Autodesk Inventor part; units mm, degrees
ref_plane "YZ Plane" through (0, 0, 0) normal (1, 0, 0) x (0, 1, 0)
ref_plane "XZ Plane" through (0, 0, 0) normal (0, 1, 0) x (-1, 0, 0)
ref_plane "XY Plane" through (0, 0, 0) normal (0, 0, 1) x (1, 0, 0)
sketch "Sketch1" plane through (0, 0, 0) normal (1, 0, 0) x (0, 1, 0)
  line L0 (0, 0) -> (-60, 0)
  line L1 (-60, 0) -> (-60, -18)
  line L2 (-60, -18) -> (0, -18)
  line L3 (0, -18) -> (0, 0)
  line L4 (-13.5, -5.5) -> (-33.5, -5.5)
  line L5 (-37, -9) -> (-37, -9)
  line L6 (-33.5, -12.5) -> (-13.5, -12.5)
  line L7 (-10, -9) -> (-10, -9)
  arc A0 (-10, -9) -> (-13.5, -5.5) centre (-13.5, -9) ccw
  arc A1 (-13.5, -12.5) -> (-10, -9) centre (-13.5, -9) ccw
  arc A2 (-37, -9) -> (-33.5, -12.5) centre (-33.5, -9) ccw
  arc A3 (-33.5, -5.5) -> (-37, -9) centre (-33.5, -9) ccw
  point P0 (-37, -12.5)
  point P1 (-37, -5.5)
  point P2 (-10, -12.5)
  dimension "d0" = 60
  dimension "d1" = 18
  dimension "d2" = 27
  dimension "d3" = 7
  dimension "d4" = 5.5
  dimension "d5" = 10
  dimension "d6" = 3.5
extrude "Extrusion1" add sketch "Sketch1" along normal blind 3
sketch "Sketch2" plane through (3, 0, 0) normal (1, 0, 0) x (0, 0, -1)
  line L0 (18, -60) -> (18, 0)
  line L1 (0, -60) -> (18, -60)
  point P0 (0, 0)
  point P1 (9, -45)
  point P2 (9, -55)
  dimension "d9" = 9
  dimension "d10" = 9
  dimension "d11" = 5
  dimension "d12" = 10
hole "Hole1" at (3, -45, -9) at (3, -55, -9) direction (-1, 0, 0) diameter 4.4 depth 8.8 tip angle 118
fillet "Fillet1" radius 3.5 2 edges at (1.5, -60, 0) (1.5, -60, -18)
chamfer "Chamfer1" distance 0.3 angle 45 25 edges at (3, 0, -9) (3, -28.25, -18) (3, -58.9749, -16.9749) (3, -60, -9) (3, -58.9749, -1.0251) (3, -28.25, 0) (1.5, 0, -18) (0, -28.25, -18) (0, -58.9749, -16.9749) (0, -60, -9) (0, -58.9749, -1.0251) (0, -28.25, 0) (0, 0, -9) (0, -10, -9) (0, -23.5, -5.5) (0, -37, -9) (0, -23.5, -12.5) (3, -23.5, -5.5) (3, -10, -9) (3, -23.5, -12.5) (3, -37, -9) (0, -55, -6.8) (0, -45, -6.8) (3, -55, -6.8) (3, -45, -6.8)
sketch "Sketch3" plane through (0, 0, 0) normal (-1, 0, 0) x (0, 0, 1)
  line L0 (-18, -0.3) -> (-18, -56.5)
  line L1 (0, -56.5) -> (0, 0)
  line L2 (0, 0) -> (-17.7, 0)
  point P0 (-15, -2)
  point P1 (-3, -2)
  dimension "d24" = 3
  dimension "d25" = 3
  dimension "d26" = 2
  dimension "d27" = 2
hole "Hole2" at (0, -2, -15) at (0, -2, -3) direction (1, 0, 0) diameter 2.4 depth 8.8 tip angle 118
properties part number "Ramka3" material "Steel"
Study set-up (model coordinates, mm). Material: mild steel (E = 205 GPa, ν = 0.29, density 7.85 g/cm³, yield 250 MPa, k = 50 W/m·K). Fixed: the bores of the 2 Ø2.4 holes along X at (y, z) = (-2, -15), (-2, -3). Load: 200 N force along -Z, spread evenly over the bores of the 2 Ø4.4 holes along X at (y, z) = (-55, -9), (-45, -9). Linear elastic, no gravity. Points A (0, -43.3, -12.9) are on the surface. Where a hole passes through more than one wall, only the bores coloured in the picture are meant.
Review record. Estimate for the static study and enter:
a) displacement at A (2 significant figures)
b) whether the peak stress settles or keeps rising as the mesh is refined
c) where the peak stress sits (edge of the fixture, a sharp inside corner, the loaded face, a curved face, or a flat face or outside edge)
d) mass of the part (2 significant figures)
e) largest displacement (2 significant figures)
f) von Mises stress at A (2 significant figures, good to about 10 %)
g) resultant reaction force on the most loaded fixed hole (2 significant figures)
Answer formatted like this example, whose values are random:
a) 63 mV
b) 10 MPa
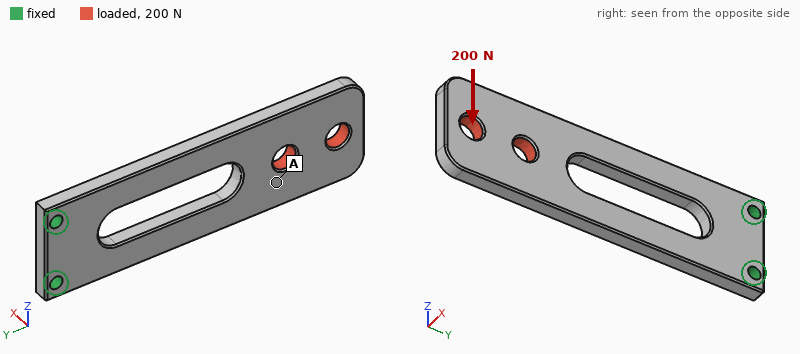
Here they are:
a) 47 µm
b) keeps rising
c) edge of the fixture
d) 20 g
e) 62 µm
f) 17 MPa
g) 730 N
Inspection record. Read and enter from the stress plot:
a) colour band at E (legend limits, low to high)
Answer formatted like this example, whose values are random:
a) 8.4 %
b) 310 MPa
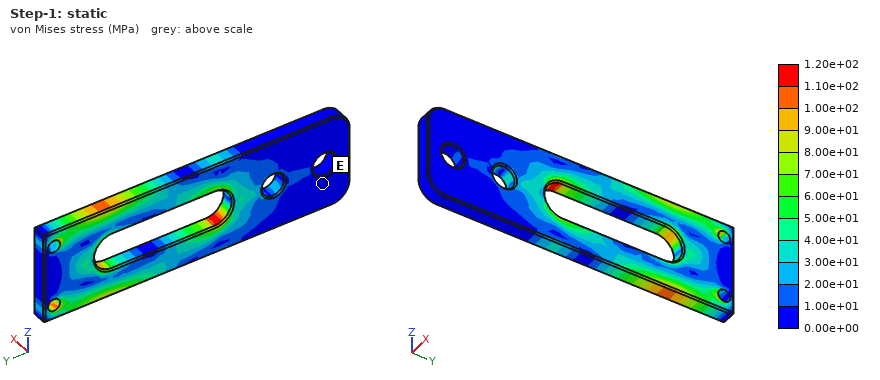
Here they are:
a) 0.00e+00 to 1.00e+01 MPa
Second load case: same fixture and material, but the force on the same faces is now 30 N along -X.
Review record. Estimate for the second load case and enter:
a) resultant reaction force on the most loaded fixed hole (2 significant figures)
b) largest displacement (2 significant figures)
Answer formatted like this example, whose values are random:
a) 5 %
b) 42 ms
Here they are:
a) 15 N
b) 0.25 mm
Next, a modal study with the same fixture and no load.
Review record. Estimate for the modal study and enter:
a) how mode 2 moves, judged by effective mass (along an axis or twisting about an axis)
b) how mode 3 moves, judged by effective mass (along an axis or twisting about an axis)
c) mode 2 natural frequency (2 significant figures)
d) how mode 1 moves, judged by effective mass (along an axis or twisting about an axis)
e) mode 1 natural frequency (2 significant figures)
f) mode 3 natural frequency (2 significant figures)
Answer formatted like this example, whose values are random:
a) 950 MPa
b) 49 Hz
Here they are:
a) along Z
b) twisting about Y
c) 3100 Hz
d) along X
e) 670 Hz
f) 3600 Hz
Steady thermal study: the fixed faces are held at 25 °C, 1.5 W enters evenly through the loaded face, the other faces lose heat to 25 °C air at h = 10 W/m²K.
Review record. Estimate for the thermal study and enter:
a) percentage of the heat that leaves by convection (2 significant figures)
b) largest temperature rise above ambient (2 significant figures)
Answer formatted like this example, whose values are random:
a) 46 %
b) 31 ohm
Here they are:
a) 25 %
b) 31 K
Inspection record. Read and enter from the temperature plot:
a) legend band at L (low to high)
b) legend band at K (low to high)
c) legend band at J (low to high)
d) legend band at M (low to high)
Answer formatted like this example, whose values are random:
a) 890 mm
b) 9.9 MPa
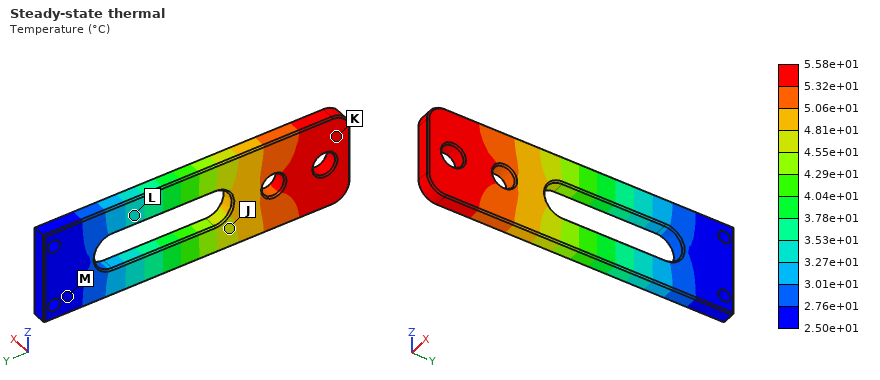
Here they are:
a) 3.27e+01 to 3.53e+01 °C
b) 5.32e+01 to 5.58e+01 °C
c) 4.55e+01 to 4.81e+01 °C
d) 2.50e+01 to 2.76e+01 °C
